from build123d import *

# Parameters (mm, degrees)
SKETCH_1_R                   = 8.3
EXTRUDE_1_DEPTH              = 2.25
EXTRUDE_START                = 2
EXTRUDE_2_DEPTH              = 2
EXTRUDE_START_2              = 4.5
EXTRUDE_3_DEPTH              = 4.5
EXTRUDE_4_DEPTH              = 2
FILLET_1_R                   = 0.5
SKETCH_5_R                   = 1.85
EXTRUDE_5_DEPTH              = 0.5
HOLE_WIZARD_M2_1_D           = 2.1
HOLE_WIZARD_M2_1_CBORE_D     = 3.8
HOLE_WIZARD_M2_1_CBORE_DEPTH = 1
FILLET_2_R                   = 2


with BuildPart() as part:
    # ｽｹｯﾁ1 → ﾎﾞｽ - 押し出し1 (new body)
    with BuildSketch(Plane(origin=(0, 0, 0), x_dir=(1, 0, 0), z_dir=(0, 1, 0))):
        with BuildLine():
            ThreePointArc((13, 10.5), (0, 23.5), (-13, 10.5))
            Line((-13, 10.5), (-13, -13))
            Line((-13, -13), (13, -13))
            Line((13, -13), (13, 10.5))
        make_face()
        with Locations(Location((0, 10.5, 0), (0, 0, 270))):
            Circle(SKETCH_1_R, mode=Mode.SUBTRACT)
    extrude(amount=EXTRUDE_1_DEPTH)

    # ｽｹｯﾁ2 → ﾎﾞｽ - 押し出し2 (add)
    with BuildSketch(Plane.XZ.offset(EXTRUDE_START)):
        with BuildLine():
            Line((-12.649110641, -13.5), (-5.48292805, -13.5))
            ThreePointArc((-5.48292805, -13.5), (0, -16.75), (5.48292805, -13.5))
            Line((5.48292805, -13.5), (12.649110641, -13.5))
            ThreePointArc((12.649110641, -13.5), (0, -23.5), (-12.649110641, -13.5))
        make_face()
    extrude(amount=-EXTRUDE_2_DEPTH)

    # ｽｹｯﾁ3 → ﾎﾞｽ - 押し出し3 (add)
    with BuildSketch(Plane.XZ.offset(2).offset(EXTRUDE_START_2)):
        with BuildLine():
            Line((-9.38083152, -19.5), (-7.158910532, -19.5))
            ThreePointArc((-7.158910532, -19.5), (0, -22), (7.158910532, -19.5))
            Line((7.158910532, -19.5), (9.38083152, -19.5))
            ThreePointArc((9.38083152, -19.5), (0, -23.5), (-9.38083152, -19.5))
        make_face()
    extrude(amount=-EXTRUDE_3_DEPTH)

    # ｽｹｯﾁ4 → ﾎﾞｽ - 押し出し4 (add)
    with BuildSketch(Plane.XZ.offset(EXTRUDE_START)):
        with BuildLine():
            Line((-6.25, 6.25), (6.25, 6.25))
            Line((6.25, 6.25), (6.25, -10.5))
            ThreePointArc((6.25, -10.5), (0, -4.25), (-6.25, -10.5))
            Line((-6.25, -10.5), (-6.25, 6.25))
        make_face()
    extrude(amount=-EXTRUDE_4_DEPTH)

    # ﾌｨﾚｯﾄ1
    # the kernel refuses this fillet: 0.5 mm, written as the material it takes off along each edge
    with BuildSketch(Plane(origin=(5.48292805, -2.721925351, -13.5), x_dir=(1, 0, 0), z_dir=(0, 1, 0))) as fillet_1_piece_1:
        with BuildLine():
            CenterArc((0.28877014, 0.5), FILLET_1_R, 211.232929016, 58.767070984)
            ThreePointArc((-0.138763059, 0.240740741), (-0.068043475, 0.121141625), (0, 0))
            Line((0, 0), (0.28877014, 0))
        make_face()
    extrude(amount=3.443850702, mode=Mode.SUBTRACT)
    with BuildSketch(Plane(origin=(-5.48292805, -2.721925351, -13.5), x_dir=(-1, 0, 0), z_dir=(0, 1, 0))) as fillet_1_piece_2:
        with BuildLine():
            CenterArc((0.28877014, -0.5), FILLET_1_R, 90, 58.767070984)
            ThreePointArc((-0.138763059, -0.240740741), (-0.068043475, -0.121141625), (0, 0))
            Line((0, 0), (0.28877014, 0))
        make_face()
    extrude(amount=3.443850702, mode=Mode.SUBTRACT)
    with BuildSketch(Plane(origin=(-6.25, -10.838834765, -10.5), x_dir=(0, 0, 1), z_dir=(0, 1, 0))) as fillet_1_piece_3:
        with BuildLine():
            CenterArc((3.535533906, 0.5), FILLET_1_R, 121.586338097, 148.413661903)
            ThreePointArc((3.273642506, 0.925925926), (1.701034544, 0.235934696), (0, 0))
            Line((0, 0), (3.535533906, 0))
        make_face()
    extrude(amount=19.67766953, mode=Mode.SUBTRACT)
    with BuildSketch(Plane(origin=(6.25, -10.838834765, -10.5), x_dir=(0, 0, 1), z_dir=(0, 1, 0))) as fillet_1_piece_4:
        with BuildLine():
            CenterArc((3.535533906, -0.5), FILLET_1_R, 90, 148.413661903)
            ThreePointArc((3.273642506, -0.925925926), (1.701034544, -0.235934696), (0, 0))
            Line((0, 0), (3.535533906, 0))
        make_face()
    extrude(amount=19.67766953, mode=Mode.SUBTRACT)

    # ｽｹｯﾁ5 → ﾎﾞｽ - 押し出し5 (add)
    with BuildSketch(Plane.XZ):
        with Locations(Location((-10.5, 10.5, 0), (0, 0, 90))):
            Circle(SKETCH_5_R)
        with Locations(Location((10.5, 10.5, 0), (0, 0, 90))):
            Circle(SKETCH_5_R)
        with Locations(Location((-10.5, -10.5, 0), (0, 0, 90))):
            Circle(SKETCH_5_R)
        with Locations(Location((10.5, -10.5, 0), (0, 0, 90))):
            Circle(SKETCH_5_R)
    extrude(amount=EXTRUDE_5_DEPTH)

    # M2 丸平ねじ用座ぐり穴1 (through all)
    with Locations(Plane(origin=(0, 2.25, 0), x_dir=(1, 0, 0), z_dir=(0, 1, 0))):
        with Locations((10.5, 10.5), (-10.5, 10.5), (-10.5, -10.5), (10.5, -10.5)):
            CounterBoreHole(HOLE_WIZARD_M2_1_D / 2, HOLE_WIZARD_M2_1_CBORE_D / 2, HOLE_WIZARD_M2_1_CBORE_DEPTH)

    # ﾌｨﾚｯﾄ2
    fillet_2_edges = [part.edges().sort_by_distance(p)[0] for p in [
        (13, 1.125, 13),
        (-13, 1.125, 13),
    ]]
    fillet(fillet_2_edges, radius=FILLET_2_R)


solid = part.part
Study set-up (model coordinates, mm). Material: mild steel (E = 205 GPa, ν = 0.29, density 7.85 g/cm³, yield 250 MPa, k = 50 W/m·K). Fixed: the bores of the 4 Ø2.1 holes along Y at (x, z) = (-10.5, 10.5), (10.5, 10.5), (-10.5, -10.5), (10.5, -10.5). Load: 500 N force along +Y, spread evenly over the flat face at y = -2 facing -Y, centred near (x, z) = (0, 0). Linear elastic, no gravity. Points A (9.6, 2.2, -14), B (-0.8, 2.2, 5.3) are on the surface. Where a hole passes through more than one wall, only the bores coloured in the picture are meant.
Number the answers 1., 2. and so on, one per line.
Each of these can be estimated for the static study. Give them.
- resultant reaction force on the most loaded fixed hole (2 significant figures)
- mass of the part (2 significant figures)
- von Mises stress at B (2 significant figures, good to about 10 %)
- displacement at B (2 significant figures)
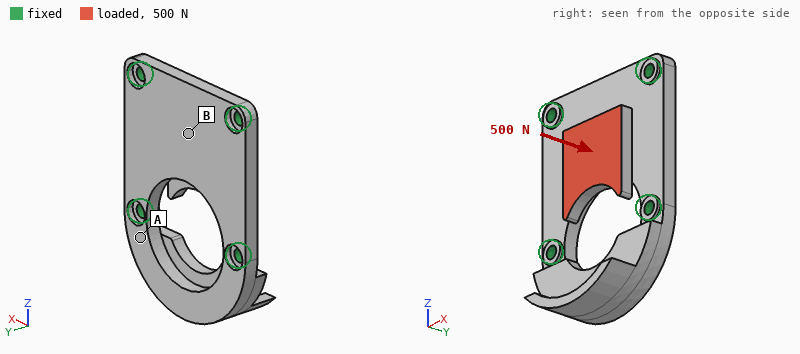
1. 170 N
2. 17 g
3. 30 MPa
4. 7.2 µm
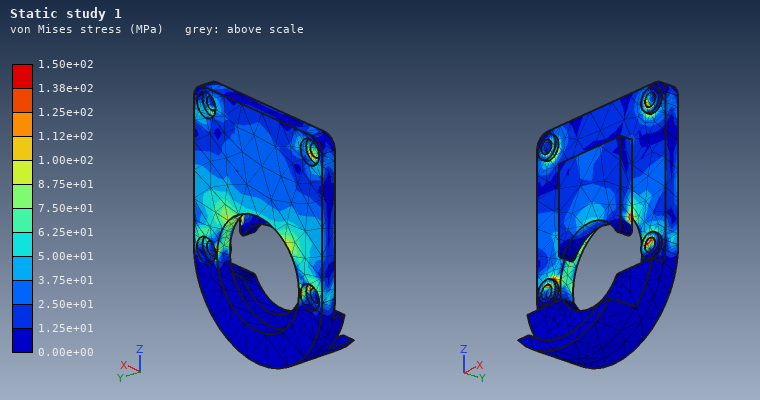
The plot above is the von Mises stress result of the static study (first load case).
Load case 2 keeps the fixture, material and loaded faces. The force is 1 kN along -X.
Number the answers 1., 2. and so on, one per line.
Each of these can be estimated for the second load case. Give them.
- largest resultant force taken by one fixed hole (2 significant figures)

1. 420 N
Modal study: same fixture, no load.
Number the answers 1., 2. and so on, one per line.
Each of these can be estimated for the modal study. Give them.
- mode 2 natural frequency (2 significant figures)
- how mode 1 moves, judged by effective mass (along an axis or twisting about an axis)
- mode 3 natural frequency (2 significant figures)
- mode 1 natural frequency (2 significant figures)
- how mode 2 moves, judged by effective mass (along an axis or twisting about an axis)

1. 15 kHz
2. along Y
3. 21 kHz
4. 4900 Hz
5. along Y
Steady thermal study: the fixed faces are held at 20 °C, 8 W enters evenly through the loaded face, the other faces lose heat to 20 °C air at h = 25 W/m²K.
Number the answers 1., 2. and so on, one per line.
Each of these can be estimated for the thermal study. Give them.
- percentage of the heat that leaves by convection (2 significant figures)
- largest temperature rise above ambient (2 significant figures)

1. 5.8 %
2. 30 K
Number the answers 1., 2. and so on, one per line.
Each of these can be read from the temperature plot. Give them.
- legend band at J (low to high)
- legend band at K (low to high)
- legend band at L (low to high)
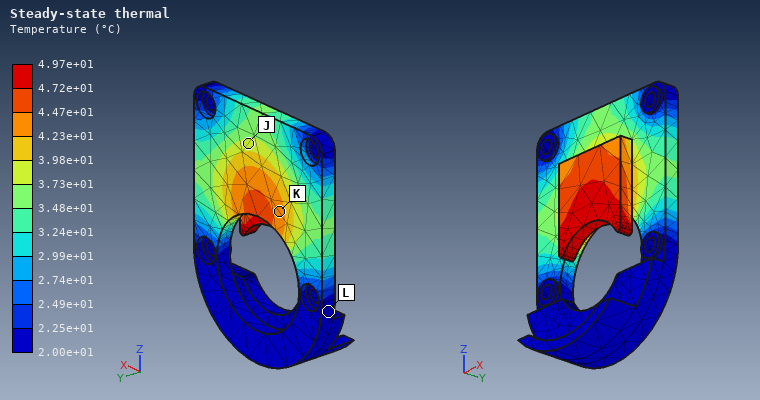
1. 3.73e+01 to 3.98e+01 °C
2. 4.23e+01 to 4.47e+01 °C
3. 2.00e+01 to 2.25e+01 °C
